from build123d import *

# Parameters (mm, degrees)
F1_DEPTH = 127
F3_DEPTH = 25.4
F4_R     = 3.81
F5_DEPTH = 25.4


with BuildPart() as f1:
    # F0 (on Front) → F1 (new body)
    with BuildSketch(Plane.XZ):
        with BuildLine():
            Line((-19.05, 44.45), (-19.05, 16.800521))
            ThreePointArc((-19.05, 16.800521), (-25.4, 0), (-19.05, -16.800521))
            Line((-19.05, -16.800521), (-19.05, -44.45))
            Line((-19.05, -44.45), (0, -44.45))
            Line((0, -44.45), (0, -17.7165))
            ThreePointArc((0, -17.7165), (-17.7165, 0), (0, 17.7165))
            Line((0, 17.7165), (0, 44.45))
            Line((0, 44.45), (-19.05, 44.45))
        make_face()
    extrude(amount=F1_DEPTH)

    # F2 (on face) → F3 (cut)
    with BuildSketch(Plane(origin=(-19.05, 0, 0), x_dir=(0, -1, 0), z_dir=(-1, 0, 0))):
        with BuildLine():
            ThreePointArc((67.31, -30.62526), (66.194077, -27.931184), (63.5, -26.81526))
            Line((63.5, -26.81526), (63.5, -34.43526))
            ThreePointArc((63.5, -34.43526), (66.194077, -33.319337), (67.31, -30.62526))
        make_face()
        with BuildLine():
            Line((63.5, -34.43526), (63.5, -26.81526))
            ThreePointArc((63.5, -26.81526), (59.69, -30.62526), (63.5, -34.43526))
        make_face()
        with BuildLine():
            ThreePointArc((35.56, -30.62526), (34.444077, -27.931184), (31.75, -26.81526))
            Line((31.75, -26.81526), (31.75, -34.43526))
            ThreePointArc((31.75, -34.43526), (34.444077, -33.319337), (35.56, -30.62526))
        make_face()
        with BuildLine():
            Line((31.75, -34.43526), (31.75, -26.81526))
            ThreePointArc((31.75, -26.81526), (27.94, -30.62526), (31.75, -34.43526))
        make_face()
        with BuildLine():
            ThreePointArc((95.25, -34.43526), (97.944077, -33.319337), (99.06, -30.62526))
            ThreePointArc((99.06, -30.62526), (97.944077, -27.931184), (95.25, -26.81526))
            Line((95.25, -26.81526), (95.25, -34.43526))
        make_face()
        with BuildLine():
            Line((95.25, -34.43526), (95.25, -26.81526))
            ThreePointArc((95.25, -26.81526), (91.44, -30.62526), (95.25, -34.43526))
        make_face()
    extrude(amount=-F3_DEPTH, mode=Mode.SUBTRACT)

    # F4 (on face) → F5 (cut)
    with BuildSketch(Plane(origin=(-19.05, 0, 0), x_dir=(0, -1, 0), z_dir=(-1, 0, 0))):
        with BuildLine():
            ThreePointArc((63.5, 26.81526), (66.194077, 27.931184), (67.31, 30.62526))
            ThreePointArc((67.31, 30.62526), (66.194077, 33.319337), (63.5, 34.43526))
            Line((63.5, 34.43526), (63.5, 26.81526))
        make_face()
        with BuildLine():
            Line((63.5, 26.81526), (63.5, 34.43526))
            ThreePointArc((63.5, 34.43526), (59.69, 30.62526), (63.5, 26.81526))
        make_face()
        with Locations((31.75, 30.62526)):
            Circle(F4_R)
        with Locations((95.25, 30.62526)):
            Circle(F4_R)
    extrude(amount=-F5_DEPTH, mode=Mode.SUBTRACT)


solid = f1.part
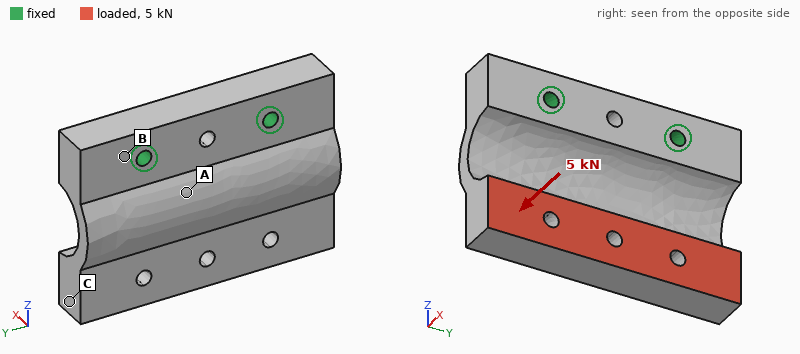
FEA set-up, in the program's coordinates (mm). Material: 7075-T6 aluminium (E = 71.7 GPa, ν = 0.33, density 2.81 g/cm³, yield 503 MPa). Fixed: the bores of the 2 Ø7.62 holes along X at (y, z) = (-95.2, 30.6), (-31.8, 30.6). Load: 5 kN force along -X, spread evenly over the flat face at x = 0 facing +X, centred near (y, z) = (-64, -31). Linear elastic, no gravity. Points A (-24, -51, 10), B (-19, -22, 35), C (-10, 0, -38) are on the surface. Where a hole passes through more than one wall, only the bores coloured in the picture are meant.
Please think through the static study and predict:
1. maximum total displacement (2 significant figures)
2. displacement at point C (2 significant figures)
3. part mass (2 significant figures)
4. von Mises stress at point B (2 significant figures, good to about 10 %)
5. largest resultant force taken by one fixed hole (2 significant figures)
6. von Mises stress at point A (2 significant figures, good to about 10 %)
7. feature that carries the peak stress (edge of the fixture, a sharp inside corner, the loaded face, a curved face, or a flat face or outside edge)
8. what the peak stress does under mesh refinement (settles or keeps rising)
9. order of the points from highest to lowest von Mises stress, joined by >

0.93 mm
0.77 mm
470 g
31 MPa
2.5 kN
120 MPa
edge of the fixture
keeps rising
A > B > C
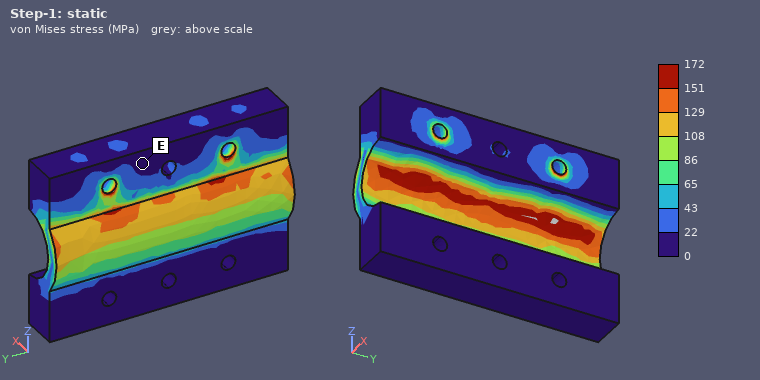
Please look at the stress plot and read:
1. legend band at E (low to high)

0 to 22 MPa
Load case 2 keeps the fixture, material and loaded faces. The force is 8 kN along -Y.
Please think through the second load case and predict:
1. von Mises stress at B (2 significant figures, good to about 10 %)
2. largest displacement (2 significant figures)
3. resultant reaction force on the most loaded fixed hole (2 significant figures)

37 MPa
0.22 mm
8.0 kN
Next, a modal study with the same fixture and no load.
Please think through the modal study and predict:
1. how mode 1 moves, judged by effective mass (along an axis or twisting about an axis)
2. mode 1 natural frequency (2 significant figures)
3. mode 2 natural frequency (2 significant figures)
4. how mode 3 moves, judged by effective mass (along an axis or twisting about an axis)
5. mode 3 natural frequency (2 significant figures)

along X
970 Hz
2100 Hz
along Y
4100 Hz
